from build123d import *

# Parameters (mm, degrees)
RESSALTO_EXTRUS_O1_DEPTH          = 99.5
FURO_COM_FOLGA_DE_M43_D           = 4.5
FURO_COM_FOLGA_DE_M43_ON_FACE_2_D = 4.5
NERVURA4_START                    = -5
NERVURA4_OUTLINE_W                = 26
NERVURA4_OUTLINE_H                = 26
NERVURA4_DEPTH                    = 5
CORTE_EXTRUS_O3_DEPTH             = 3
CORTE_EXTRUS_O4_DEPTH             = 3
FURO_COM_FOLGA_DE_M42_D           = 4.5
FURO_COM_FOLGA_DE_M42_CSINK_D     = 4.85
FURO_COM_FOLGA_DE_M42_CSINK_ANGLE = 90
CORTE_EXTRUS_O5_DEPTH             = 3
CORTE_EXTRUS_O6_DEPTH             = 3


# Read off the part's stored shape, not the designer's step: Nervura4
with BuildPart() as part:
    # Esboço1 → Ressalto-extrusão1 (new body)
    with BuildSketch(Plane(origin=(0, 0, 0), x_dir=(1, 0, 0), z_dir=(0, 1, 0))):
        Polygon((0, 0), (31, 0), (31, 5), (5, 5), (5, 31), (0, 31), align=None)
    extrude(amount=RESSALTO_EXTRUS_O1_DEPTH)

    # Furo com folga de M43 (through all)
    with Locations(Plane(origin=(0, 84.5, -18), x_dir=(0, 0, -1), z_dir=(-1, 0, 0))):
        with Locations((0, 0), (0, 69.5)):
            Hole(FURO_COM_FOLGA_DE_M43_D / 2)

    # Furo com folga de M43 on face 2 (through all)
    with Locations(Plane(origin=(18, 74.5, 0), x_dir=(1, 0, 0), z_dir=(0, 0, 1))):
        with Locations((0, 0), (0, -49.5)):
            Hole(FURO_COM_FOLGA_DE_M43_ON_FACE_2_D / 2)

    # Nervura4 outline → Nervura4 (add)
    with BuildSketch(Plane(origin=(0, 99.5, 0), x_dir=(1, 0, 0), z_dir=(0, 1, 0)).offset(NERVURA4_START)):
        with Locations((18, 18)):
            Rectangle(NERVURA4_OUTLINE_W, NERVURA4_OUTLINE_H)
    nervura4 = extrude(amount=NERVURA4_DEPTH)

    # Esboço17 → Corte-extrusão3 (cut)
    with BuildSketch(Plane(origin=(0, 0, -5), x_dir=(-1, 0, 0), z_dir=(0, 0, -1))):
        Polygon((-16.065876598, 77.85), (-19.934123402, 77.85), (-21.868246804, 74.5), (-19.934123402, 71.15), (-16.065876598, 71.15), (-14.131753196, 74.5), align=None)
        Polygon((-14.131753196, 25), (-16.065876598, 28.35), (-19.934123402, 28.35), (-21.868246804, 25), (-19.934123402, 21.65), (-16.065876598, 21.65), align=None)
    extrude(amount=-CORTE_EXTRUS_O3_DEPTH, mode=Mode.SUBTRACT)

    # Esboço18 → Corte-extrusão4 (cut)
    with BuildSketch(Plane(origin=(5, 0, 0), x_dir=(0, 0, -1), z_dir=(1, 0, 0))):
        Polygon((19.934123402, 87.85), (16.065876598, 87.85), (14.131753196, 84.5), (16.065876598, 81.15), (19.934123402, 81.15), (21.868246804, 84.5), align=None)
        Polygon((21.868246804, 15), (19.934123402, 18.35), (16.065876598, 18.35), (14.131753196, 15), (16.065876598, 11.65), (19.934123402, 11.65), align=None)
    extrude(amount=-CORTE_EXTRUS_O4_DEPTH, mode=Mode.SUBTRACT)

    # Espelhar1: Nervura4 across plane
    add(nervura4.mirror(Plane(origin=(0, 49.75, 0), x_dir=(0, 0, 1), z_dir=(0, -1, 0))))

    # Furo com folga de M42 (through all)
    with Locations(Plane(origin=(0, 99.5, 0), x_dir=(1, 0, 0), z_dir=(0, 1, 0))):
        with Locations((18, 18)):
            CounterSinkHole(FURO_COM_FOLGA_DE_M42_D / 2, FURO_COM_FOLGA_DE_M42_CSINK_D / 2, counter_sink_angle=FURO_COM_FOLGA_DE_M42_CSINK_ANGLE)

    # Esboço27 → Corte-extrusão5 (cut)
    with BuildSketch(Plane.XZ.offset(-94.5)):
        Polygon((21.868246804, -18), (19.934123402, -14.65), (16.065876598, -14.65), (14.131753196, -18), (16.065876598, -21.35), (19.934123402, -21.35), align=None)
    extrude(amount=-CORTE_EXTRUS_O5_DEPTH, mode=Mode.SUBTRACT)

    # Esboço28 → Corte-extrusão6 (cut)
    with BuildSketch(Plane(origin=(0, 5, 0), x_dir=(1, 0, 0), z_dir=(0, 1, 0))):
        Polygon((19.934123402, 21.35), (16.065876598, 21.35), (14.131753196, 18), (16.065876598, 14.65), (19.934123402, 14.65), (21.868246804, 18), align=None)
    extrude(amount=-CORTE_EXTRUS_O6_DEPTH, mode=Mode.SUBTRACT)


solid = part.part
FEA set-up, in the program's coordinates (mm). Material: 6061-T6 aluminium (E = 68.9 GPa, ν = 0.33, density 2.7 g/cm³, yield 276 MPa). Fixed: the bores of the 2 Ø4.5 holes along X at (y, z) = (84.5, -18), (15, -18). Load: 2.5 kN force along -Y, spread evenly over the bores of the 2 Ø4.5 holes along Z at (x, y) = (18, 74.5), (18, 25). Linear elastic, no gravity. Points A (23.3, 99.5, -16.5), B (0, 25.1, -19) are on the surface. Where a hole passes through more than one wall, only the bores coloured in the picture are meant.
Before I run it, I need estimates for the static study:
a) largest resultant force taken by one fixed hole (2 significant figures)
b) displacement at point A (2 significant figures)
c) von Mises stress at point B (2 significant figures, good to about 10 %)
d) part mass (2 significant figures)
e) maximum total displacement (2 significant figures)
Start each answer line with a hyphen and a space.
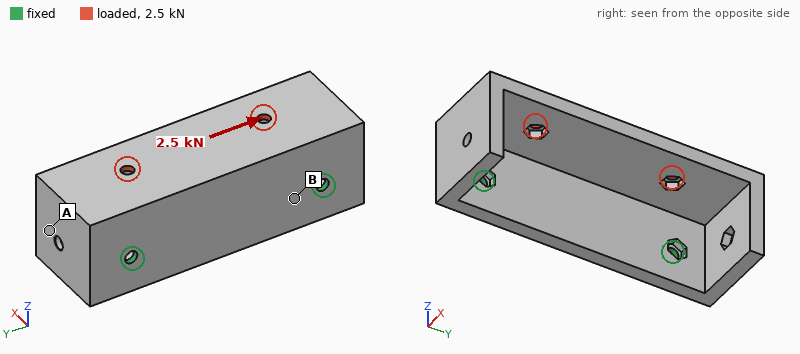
- 1.5 kN
- 61 µm
- 18 MPa
- 92 g
- 95 µm
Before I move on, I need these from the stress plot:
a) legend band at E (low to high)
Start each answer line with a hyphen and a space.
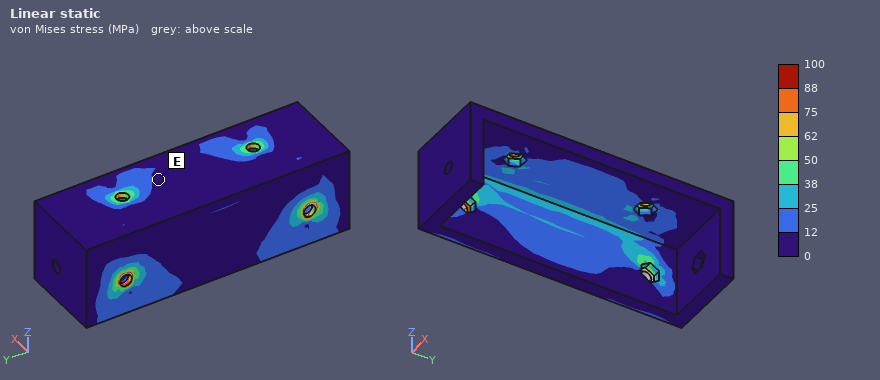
- 0 to 12 MPa
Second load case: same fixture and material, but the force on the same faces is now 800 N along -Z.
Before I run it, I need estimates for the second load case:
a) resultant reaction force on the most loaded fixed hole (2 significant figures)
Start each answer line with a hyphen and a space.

- 410 N
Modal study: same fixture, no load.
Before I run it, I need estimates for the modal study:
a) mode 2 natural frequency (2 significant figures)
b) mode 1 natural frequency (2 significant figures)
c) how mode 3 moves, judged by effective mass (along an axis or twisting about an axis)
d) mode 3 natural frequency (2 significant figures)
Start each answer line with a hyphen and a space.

- 2400 Hz
- 1400 Hz
- along X
- 5100 Hz
